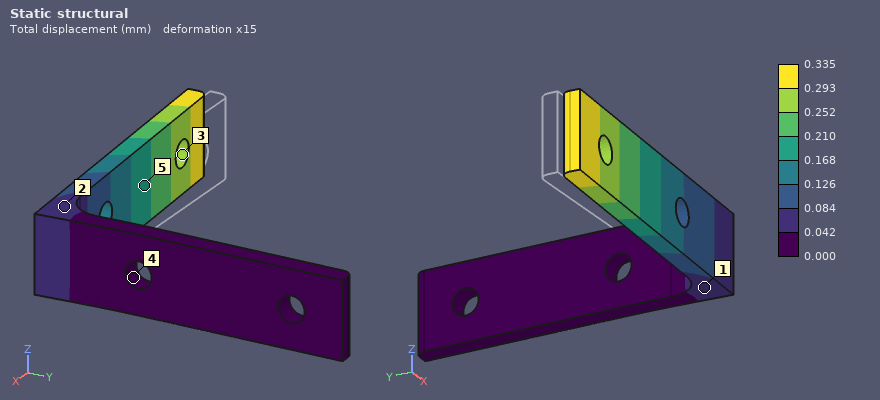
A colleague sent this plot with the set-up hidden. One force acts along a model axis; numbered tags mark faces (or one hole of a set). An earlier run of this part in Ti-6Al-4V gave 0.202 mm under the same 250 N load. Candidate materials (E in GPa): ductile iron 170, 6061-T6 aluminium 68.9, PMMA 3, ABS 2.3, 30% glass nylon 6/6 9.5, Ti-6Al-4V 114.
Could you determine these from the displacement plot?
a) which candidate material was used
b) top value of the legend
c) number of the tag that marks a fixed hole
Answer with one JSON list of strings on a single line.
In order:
["6061-T6 aluminium", "0.335 mm", "4"]
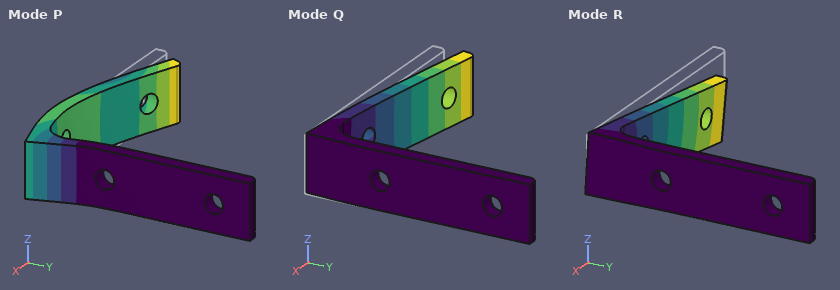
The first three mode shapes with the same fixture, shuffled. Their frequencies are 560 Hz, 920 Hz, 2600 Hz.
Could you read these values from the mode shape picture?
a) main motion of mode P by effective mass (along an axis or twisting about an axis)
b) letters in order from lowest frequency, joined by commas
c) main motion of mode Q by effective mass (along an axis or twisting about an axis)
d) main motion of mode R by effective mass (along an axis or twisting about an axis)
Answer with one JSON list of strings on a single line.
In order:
["along X", "Q, R, P", "along Y", "along Z"]
